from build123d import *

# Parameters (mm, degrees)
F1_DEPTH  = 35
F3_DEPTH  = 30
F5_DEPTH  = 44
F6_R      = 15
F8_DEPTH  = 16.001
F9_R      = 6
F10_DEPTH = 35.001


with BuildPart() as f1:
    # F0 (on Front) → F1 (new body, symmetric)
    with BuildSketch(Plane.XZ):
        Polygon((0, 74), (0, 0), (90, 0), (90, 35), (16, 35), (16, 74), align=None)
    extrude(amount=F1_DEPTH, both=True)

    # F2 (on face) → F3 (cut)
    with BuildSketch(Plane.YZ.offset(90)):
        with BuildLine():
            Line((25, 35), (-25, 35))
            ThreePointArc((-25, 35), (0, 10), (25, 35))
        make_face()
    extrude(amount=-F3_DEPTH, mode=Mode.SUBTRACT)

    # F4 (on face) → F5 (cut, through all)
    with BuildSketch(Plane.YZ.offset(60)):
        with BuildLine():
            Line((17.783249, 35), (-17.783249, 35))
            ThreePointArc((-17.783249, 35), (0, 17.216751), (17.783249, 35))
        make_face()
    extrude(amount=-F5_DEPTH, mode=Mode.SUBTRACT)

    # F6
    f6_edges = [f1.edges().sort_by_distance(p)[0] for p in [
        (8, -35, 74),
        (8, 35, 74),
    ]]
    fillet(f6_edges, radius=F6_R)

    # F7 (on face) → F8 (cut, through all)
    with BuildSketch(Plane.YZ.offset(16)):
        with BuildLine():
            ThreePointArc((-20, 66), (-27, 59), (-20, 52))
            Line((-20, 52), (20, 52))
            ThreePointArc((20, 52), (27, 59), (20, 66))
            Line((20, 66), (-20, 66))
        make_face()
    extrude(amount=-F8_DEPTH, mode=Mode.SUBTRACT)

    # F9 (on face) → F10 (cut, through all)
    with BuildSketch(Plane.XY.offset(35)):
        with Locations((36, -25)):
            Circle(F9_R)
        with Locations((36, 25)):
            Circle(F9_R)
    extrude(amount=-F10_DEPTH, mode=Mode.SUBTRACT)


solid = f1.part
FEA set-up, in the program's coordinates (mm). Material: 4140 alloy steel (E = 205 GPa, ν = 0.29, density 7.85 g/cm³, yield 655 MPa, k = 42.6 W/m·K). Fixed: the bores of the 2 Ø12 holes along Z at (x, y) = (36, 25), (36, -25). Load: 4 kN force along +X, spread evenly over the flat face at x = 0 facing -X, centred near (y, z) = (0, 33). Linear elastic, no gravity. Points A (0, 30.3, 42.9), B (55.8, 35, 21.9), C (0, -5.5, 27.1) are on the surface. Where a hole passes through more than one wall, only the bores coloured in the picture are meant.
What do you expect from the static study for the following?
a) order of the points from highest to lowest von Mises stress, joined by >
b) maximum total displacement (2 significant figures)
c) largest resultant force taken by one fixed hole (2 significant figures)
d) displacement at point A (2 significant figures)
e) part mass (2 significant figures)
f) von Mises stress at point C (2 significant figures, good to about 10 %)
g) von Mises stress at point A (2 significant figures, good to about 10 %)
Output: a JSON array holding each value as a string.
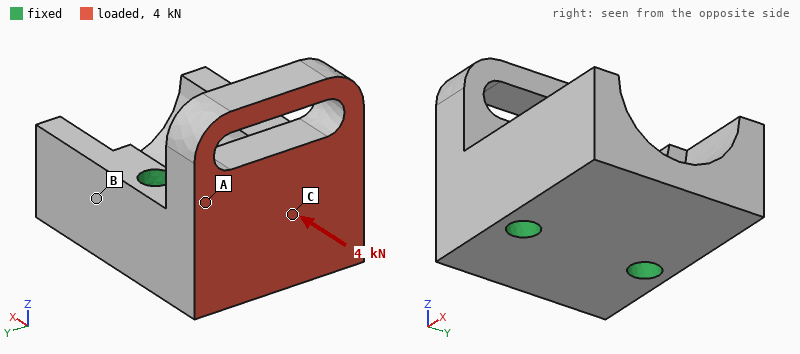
["A > C > B", "14 µm", "2.0 kN", "3.5 µm", "1.5 kg", "6.6 MPa", "12 MPa"]
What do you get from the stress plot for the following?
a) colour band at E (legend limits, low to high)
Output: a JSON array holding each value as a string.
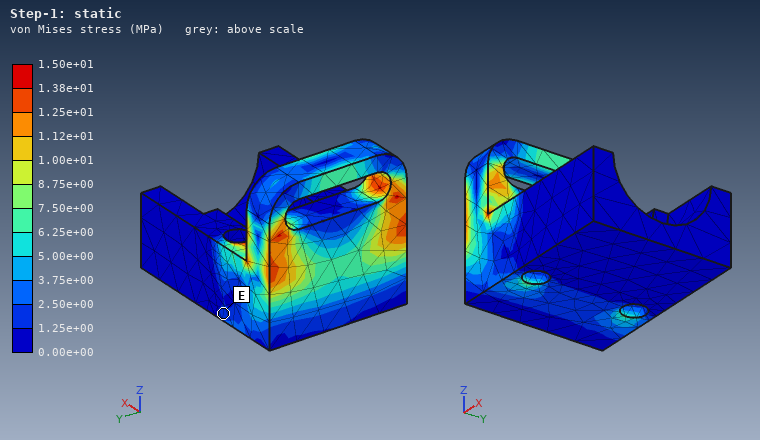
["1.25e+00 to 2.50e+00 MPa"]
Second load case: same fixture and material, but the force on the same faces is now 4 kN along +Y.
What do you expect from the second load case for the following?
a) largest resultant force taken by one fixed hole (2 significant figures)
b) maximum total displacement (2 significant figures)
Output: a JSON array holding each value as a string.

["3.1 kN", "6.4 µm"]
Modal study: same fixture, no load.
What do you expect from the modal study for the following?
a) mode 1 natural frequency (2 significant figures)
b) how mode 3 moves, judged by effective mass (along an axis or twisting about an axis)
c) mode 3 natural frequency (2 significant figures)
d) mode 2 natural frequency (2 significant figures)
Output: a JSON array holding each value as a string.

["4600 Hz", "twisting about Y", "8500 Hz", "6600 Hz"]
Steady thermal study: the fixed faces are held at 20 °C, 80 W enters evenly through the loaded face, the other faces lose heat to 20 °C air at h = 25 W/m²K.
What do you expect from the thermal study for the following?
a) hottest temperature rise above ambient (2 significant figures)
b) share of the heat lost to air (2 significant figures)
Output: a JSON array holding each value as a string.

["56 K", "11 %"]
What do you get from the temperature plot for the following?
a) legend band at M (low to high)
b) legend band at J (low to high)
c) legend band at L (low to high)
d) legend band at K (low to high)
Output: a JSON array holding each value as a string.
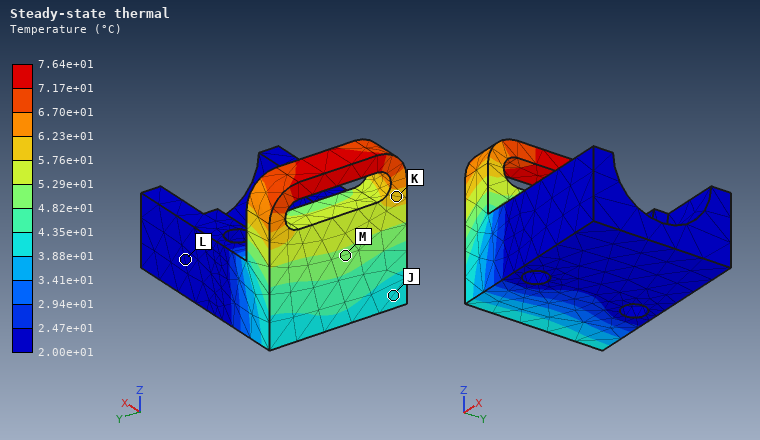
["4.82e+01 to 5.29e+01 °C", "3.88e+01 to 4.35e+01 °C", "2.00e+01 to 2.47e+01 °C", "5.76e+01 to 6.23e+01 °C"]
